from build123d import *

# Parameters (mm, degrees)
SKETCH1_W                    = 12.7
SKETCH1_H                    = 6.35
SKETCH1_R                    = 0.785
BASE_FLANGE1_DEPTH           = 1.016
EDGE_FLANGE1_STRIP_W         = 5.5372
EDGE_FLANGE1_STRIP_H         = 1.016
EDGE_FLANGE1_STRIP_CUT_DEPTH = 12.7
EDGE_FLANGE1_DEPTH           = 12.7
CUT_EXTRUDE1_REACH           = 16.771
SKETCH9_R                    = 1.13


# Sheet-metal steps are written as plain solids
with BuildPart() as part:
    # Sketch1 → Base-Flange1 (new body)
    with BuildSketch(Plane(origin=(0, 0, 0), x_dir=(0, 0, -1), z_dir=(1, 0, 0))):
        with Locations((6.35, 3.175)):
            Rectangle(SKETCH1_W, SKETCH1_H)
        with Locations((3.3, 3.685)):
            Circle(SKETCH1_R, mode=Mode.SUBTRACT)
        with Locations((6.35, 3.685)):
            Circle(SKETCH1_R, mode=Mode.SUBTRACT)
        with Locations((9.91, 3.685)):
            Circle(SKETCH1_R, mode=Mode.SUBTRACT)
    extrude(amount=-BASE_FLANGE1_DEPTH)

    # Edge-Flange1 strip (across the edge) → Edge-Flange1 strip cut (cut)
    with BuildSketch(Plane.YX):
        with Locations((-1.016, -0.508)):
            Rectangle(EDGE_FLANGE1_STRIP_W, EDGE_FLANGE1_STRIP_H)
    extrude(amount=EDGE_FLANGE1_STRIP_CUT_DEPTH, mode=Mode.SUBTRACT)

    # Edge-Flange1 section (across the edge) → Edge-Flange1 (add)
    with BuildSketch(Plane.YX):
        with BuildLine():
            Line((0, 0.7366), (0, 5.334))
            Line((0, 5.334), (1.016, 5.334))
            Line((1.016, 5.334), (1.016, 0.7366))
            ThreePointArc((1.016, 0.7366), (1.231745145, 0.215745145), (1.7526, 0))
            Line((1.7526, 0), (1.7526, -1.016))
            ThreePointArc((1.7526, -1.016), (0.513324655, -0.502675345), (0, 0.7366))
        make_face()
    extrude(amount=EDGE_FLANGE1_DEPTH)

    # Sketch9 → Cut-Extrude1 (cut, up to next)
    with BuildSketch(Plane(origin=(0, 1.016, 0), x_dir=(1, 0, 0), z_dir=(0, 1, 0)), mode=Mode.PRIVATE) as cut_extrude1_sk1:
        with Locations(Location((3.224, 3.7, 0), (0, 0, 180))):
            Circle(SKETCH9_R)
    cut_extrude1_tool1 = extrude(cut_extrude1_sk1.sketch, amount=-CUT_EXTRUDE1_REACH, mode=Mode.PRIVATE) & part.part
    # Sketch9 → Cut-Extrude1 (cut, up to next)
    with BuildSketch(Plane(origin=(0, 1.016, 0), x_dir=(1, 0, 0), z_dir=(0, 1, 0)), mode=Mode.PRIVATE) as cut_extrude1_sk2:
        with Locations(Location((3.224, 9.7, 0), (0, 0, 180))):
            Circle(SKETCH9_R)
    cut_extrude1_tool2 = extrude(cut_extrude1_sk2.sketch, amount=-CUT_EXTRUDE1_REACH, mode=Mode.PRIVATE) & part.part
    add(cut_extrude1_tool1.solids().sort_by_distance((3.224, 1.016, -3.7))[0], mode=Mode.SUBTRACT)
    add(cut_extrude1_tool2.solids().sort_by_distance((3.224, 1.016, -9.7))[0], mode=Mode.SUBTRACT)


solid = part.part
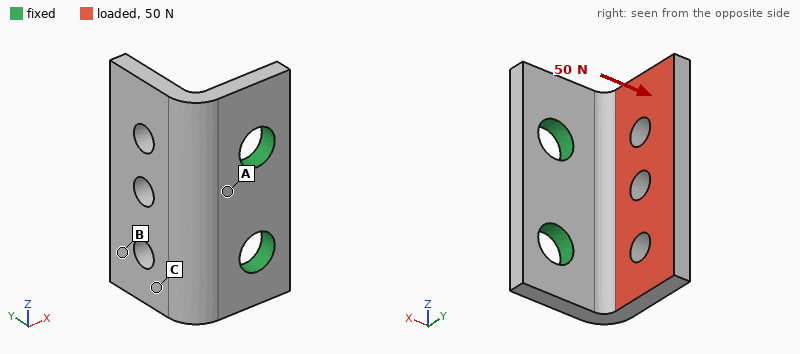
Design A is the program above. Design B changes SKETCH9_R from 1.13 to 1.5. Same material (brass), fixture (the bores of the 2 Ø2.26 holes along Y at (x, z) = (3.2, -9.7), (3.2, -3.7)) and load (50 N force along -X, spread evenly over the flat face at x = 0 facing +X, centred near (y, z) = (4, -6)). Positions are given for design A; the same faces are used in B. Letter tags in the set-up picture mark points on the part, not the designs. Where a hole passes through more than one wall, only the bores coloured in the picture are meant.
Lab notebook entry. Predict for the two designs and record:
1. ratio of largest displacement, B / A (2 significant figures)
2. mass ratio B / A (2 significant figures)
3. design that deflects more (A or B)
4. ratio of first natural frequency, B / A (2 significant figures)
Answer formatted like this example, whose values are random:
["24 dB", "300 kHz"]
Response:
["0.89", "0.95", "A", "1.1"]
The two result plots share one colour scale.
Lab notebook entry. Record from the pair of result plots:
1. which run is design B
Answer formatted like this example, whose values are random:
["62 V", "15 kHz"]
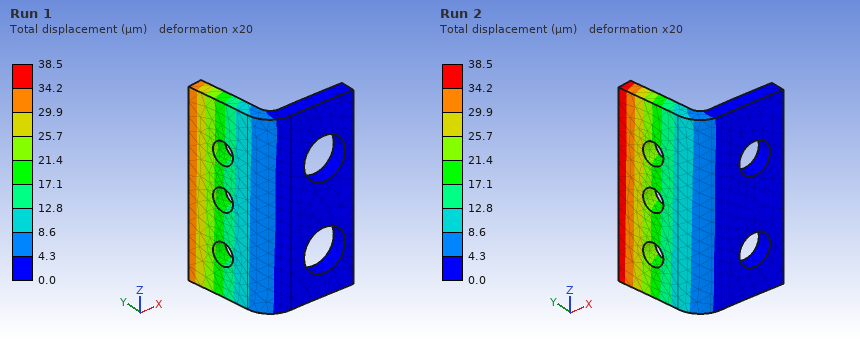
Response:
["Run 1"]
